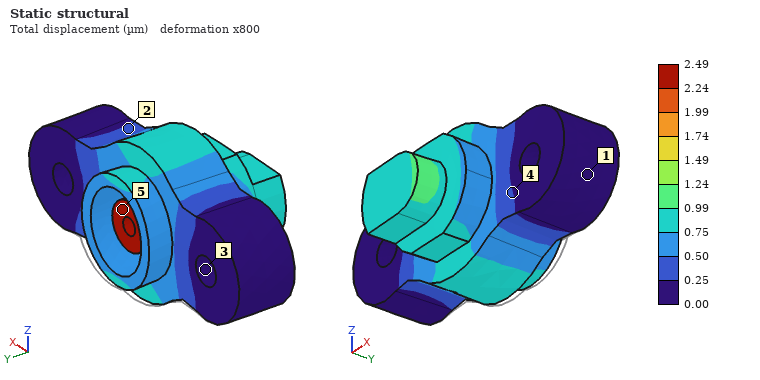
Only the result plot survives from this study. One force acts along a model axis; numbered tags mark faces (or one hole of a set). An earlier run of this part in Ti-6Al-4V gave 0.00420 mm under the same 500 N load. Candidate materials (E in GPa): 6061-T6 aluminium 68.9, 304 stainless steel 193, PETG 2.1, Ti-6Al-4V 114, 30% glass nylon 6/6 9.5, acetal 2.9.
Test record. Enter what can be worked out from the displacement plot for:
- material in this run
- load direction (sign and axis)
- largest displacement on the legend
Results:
304 stainless steel
-Y
2.49 µm
